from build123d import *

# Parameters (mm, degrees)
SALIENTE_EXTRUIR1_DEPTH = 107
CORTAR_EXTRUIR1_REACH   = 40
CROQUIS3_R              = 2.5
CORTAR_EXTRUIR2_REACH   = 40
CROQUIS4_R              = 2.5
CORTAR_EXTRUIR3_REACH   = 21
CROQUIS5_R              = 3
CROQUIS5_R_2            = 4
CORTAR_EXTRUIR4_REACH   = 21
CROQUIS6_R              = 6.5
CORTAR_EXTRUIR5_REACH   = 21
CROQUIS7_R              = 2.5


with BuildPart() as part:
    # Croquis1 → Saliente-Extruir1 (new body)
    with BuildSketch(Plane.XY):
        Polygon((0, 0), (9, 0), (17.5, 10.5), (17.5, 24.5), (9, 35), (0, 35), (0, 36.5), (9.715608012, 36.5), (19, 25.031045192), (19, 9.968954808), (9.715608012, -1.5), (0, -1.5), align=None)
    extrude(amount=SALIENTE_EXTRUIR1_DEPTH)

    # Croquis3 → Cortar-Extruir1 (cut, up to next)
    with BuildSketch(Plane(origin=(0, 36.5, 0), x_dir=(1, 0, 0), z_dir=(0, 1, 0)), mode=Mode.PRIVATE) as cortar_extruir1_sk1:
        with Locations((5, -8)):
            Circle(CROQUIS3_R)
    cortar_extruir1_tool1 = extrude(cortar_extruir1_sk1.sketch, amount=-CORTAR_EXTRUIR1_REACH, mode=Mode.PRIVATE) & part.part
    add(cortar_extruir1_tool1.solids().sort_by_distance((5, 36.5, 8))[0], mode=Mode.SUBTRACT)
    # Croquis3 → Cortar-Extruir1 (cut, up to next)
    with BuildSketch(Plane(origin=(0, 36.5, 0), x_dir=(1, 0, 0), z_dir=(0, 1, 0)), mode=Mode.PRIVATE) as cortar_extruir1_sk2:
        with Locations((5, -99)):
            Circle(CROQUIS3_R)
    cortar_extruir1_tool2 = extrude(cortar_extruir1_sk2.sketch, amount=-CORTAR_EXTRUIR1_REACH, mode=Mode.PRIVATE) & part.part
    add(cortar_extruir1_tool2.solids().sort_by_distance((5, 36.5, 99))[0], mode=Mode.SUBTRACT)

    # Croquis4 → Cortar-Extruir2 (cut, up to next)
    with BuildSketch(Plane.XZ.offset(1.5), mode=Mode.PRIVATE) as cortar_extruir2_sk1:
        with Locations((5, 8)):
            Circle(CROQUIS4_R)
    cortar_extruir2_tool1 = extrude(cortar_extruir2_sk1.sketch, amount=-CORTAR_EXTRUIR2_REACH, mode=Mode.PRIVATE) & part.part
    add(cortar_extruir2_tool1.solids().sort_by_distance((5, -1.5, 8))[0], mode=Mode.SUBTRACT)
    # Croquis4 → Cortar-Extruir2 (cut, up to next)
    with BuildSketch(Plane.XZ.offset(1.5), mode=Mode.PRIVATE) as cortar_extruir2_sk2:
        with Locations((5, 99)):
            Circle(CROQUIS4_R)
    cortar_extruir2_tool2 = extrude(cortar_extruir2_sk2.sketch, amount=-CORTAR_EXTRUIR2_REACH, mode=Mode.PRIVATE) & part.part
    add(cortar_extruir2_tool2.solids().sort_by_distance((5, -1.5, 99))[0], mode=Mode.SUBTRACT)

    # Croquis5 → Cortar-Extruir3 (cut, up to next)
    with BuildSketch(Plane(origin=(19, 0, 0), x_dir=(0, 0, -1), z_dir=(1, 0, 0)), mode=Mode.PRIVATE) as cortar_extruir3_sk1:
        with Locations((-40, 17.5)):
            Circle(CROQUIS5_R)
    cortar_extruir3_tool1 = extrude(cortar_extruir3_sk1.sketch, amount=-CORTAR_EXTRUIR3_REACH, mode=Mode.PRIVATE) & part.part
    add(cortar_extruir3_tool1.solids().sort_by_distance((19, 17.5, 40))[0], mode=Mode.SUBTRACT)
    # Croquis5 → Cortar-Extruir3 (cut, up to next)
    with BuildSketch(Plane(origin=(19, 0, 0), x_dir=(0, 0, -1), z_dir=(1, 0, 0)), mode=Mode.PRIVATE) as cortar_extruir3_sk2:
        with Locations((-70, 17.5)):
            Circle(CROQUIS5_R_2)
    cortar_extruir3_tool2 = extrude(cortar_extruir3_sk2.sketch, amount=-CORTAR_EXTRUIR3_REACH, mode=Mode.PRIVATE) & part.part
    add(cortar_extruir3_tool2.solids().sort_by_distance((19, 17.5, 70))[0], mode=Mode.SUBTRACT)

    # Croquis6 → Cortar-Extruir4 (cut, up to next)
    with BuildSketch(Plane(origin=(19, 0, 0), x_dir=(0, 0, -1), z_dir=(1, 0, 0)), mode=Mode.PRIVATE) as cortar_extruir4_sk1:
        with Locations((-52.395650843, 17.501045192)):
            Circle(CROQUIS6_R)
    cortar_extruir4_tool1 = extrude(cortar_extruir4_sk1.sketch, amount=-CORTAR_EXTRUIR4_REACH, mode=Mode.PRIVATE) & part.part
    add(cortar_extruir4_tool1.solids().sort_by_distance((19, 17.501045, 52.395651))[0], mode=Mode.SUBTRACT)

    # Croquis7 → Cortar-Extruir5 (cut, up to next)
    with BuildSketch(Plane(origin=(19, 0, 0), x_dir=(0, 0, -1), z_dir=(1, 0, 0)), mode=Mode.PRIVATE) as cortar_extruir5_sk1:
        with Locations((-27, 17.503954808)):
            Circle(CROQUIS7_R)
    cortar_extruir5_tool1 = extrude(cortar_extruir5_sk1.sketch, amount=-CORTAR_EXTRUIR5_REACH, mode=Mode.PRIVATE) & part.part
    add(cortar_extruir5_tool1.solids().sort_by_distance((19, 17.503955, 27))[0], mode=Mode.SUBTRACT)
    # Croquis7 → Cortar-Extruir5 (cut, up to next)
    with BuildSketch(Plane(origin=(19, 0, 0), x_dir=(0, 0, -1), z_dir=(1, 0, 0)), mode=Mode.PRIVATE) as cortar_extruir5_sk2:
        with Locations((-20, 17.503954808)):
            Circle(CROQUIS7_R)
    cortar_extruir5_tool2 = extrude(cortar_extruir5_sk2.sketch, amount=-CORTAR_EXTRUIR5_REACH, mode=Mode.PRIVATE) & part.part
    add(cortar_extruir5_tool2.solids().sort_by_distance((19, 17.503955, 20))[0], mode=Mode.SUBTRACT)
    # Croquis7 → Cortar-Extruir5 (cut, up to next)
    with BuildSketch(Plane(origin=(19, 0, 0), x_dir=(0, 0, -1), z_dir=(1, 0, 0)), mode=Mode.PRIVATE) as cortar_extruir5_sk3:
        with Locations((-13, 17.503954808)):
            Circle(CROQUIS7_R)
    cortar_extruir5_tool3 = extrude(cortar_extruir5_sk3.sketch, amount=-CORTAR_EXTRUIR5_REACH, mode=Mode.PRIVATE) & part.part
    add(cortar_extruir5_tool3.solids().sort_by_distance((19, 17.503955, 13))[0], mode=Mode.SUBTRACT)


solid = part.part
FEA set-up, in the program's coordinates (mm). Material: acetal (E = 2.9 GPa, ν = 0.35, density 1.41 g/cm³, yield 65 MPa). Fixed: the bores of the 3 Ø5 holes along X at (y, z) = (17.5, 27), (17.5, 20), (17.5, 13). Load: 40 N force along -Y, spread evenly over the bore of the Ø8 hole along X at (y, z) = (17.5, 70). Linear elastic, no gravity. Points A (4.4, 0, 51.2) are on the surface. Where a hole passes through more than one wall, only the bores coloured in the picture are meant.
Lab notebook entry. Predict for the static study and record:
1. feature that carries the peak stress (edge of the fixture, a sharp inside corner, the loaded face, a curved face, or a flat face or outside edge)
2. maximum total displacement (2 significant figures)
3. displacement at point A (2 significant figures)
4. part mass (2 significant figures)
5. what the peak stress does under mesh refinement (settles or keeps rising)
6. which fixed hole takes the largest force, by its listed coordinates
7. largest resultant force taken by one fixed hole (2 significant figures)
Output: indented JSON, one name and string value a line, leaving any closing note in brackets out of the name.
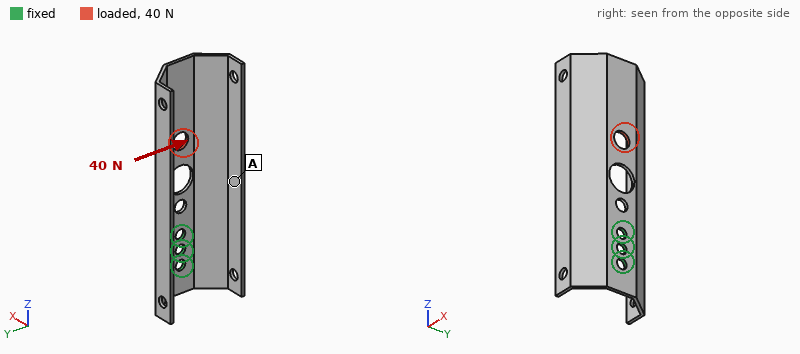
{
  "feature that carries the peak stress": "edge of the fixture",
  "maximum total displacement": "1.1 mm",
  "displacement at point A": "0.35 mm",
  "part mass": "13 g",
  "what the peak stress does under mesh refinement": "keeps rising",
  "which fixed hole takes the largest force, by its listed coordinates": "(17.5, 27)",
  "largest resultant force taken by one fixed hole": "120 N"
}
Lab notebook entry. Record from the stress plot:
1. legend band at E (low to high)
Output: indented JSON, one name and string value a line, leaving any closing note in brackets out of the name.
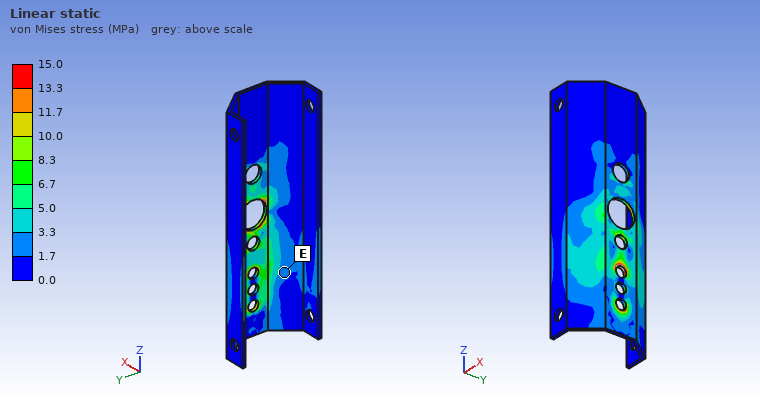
{
  "legend band at E": "1.7 to 3.3 MPa"
}
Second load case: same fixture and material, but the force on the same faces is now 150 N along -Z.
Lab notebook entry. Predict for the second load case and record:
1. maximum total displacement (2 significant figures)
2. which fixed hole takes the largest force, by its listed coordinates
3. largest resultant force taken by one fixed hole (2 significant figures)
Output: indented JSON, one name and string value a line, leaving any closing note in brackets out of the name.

{
  "maximum total displacement": "0.64 mm",
  "which fixed hole takes the largest force, by its listed coordinates": "(17.5, 27)",
  "largest resultant force taken by one fixed hole": "97 N"
}
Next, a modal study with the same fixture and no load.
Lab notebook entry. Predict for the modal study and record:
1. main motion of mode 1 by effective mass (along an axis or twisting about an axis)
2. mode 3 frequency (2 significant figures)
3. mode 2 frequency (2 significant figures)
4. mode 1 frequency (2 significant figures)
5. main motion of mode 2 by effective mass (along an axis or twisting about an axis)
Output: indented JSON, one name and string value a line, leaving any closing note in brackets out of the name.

{
  "main motion of mode 1 by effective mass": "along Y",
  "mode 3 frequency": "470 Hz",
  "mode 2 frequency": "200 Hz",
  "mode 1 frequency": "150 Hz",
  "main motion of mode 2 by effective mass": "along X"
}
